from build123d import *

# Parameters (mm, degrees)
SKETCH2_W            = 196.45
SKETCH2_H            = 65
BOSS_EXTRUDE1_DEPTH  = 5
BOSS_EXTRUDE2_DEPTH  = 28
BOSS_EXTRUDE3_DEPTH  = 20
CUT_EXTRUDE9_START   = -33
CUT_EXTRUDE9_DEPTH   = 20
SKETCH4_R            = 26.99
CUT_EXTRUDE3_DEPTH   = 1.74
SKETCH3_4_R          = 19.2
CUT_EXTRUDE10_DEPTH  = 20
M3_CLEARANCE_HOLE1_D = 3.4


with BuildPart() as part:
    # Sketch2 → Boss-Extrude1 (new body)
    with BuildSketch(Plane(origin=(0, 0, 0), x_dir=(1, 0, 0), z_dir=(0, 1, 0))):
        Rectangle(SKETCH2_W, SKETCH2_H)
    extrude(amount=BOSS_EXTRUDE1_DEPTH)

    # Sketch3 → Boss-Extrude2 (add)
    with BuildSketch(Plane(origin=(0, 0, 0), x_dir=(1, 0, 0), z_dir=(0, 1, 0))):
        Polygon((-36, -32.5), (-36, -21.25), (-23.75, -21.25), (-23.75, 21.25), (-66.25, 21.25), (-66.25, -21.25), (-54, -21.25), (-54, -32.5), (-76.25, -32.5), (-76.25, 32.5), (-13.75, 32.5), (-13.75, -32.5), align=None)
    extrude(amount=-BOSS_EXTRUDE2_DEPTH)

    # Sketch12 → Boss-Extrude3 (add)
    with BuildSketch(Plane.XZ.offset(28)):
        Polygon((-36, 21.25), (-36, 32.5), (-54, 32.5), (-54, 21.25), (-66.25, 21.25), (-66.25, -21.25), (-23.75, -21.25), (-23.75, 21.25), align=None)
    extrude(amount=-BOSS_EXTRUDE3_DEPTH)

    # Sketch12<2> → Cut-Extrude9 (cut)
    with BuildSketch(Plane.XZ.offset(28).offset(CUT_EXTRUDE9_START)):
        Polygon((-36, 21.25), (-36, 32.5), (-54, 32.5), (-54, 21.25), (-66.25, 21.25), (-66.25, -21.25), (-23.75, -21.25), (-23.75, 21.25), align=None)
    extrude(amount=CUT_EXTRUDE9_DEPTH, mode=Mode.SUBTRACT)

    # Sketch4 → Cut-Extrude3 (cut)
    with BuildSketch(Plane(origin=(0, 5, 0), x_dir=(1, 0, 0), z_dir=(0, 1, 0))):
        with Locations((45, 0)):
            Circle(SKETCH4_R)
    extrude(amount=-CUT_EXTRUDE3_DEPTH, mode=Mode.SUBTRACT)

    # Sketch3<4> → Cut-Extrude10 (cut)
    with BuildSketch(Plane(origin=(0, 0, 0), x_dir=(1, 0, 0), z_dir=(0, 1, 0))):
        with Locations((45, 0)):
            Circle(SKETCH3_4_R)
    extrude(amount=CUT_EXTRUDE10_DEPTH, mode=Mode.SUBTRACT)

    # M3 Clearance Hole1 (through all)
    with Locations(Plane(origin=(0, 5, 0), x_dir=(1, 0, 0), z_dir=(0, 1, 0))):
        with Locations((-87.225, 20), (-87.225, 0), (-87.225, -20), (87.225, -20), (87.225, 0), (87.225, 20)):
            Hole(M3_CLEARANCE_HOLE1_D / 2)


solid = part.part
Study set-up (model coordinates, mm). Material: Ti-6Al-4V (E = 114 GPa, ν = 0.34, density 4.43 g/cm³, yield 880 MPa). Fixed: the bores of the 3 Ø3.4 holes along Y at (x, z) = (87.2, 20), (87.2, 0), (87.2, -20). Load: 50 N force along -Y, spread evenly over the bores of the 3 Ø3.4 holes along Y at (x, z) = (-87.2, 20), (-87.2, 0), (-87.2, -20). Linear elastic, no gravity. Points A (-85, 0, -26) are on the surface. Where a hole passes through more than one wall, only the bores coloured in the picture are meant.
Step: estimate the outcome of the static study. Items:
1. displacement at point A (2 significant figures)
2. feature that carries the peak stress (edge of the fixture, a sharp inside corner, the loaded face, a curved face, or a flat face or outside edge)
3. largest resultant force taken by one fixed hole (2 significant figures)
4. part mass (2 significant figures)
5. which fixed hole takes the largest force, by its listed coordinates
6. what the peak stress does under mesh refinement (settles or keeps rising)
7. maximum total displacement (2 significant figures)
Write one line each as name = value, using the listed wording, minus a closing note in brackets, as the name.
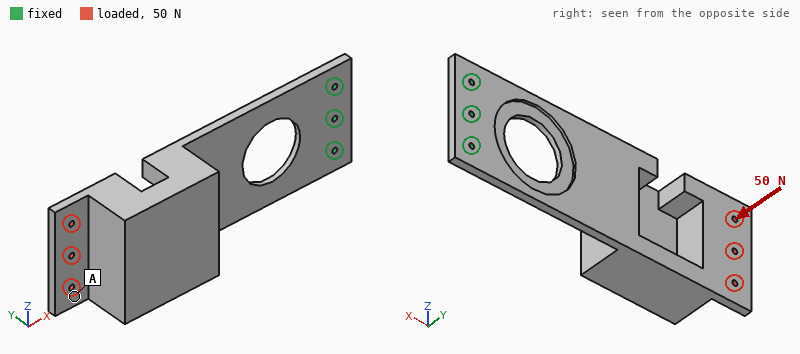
displacement at point A = 2.1 mm
feature that carries the peak stress = a sharp inside corner
largest resultant force taken by one fixed hole = 140 N
part mass = 570 g
which fixed hole takes the largest force, by its listed coordinates = (87.2, 0)
what the peak stress does under mesh refinement = keeps rising
maximum total displacement = 2.3 mm
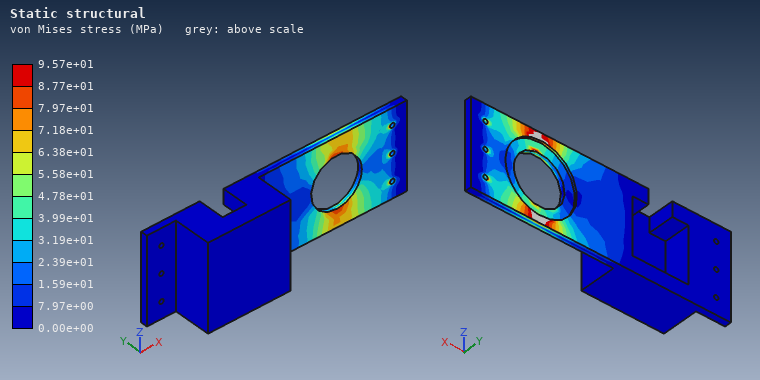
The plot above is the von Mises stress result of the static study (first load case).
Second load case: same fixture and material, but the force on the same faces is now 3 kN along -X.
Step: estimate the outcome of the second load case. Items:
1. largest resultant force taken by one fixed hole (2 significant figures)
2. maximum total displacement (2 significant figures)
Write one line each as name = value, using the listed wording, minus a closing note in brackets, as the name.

largest resultant force taken by one fixed hole = 1.4 kN
maximum total displacement = 0.38 mm
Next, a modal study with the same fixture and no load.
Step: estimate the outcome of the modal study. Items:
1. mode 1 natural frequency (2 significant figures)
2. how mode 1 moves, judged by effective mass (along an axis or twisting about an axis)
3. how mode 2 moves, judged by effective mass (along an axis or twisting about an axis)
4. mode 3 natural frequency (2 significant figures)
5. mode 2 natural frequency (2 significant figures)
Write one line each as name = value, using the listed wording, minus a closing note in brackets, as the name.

mode 1 natural frequency = 49 Hz
how mode 1 moves, judged by effective mass = along Y
how mode 2 moves, judged by effective mass = along Z
mode 3 natural frequency = 550 Hz
mode 2 natural frequency = 250 Hz
